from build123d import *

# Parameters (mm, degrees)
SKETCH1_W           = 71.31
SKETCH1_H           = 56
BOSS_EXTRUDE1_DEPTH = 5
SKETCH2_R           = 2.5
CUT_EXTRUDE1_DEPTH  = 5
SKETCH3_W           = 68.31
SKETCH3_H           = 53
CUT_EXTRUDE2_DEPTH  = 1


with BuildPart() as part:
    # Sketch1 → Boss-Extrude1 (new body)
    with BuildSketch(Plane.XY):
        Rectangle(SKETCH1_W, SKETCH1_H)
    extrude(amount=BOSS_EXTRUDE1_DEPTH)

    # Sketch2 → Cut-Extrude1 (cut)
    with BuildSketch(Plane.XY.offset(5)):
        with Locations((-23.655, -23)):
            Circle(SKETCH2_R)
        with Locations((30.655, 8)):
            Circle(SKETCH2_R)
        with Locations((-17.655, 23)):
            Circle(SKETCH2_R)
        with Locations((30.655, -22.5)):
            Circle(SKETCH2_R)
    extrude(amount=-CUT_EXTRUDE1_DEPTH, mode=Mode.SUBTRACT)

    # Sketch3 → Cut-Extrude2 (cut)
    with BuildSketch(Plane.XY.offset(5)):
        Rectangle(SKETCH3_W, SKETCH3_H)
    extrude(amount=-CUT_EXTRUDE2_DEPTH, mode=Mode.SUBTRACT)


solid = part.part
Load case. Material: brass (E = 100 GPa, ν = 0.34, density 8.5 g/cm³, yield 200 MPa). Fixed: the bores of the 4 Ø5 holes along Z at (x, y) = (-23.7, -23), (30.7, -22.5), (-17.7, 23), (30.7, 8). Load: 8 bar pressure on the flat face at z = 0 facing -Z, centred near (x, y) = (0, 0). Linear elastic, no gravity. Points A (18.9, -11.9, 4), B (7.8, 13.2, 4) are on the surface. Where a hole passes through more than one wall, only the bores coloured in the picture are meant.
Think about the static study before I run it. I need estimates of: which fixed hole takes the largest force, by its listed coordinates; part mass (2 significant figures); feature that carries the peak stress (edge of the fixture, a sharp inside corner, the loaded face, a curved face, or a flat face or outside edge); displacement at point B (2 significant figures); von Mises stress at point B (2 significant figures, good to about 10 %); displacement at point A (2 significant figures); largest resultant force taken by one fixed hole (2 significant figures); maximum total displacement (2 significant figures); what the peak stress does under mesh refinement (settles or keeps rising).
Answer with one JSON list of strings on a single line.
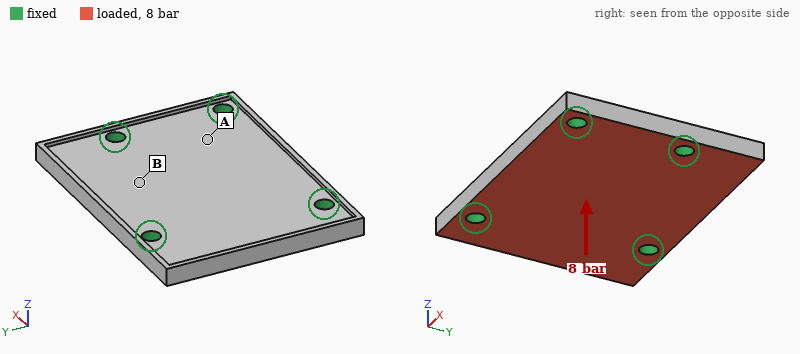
["(-17.7, 23)", "140 g", "edge of the fixture", "31 µm", "33 MPa", "20 µm", "960 N", "38 µm", "keeps rising"]
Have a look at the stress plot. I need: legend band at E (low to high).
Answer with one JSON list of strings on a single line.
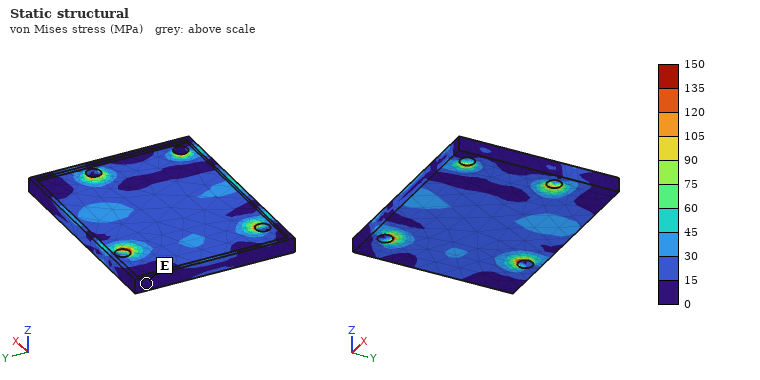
["0 to 15 MPa"]
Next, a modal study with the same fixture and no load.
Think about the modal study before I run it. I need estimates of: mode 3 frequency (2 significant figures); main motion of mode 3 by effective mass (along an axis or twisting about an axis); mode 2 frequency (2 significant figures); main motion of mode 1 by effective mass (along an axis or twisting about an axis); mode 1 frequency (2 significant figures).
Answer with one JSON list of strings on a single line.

["5500 Hz", "along Z", "5100 Hz", "along Z", "4600 Hz"]
